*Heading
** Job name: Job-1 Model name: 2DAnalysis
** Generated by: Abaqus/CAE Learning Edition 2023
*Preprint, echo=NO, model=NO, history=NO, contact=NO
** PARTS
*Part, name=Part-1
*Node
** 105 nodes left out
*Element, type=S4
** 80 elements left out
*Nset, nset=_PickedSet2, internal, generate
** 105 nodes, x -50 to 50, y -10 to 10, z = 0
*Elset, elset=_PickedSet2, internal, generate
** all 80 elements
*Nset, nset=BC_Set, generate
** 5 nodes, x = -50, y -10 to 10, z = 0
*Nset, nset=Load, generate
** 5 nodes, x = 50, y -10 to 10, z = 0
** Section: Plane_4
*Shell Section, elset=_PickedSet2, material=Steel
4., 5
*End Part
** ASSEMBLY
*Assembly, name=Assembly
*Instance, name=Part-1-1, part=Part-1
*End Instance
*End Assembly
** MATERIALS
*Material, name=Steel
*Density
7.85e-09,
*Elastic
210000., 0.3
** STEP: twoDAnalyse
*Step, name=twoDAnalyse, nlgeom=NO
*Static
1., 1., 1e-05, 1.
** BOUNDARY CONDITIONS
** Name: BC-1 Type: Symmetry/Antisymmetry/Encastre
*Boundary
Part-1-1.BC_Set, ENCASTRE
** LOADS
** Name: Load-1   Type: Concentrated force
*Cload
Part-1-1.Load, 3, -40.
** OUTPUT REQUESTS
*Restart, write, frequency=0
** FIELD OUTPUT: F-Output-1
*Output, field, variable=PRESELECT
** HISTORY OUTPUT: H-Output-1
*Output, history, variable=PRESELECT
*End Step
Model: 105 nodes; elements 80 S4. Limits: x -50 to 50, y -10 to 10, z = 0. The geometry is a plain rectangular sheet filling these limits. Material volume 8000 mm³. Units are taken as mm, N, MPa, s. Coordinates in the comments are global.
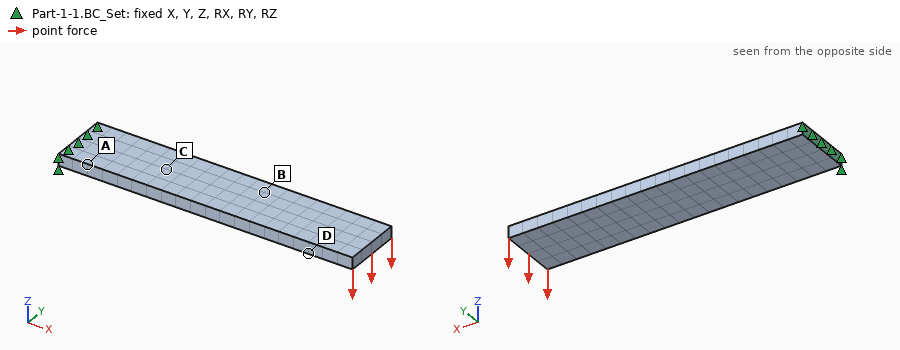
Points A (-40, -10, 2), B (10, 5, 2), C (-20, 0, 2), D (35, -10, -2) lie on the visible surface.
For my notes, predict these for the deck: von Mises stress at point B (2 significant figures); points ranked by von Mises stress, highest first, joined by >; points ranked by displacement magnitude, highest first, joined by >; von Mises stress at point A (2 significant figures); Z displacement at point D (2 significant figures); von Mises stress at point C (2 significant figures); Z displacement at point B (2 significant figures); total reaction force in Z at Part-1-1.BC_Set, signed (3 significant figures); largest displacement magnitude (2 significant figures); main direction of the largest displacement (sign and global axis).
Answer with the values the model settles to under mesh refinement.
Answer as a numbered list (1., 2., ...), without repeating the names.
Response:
1. 150 MPa
2. A > C > B > D
3. D > B > C > A
4. 340 MPa
5. -2.3 mm
6. 260 MPa
7. -1.2 mm
8. 200 N
9. 2.9 mm
10. -Z
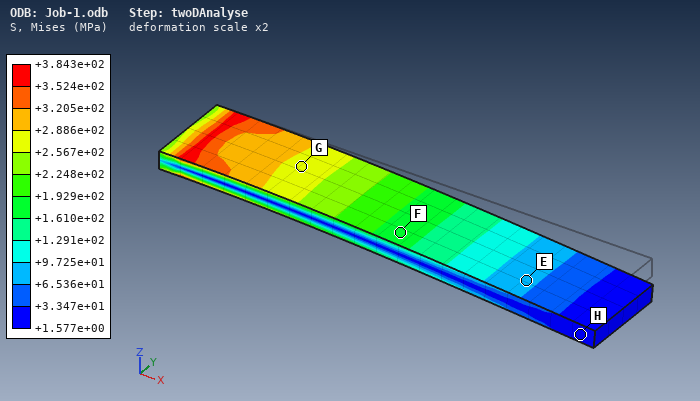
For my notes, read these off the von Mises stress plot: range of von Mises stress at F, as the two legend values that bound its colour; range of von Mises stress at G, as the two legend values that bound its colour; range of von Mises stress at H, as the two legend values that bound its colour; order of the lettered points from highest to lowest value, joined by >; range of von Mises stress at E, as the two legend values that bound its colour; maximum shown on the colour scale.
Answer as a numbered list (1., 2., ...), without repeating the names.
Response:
1. +1.610e+02 to +1.929e+02 MPa
2. +2.567e+02 to +2.886e+02 MPa
3. +1.577e+00 to +3.347e+01 MPa
4. G > F > E > H
5. +6.536e+01 to +9.725e+01 MPa
6. +3.843e+02 MPa
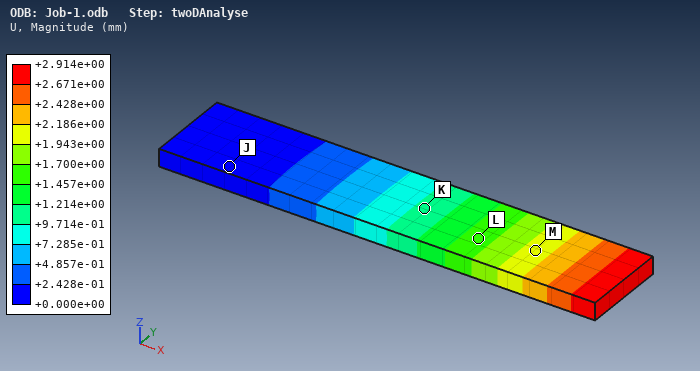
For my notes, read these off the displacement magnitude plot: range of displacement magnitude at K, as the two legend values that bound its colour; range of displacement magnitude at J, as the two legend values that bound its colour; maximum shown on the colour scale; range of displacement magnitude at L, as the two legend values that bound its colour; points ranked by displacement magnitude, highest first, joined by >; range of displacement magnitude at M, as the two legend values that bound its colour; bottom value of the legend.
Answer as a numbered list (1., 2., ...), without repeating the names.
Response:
1. +9.714e-01 to +1.214e+00 mm
2. +0.000e+00 to +2.428e-01 mm
3. +2.914e+00 mm
4. +1.457e+00 to +1.700e+00 mm
5. M > L > K > J
6. +1.943e+00 to +2.186e+00 mm
7. +0.000e+00 mm
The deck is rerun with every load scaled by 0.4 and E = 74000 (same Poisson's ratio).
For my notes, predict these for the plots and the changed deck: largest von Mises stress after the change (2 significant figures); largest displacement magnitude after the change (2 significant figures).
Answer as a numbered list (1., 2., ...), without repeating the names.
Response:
1. 150 MPa
2. 3.3 mm
